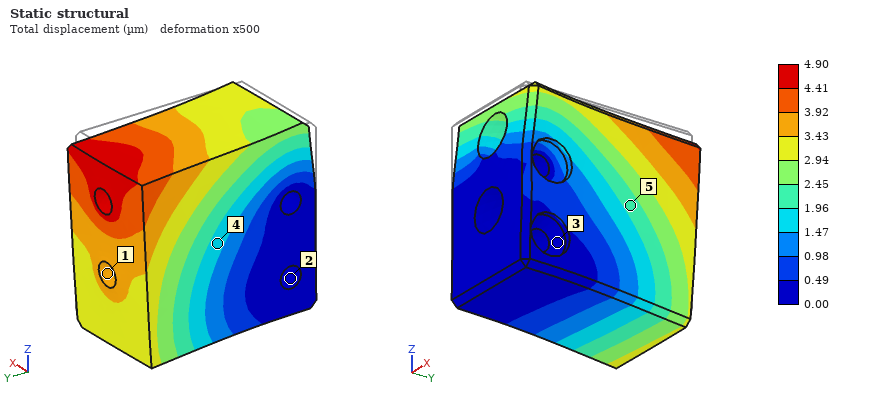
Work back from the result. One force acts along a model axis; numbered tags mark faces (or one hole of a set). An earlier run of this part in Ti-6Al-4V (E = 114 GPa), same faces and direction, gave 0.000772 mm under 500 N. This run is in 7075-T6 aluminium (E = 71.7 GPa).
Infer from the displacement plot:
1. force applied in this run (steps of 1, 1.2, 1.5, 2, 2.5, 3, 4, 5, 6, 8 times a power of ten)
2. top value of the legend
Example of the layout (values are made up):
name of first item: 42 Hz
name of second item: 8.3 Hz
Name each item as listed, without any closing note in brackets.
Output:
force applied in this run: 2 kN
top value of the legend: 4.90 µm
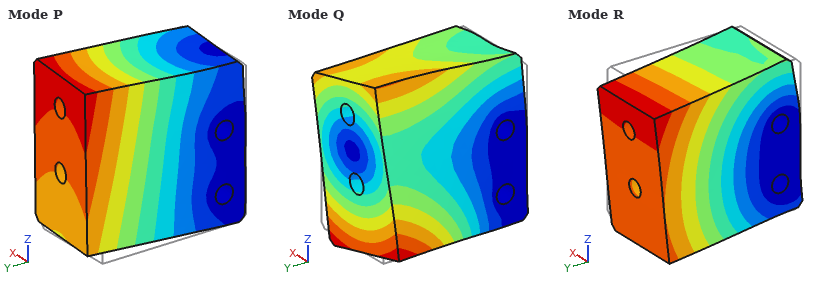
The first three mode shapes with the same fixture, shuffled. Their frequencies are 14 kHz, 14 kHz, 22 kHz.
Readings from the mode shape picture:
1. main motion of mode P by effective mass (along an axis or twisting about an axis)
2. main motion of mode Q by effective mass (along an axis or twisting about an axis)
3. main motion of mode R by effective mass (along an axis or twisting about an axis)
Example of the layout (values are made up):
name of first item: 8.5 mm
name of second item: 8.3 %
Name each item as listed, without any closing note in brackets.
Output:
main motion of mode P by effective mass: along X
main motion of mode Q by effective mass: twisting about Y
main motion of mode R by effective mass: along Z
